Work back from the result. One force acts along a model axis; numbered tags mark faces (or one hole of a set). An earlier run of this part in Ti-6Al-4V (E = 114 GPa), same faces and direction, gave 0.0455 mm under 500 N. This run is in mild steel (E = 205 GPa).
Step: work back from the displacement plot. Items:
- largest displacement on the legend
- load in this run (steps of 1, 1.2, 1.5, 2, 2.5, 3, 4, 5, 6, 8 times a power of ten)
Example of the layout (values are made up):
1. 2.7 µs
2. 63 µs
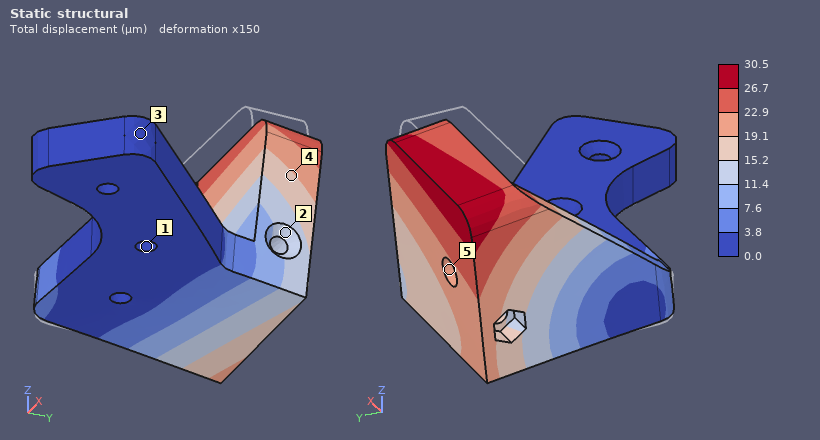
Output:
1. 30.5 µm
2. 600 N
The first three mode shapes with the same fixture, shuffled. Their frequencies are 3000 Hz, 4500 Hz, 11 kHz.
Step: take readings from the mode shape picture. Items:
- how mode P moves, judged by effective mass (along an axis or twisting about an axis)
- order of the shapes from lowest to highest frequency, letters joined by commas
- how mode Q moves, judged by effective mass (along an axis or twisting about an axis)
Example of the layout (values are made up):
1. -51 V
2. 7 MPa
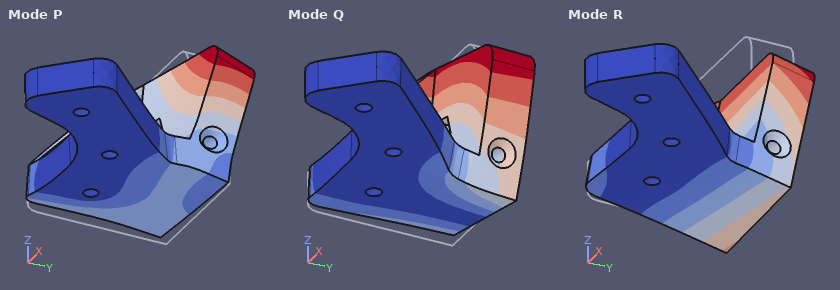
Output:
1. along Z
2. R, Q, P
3. along X
